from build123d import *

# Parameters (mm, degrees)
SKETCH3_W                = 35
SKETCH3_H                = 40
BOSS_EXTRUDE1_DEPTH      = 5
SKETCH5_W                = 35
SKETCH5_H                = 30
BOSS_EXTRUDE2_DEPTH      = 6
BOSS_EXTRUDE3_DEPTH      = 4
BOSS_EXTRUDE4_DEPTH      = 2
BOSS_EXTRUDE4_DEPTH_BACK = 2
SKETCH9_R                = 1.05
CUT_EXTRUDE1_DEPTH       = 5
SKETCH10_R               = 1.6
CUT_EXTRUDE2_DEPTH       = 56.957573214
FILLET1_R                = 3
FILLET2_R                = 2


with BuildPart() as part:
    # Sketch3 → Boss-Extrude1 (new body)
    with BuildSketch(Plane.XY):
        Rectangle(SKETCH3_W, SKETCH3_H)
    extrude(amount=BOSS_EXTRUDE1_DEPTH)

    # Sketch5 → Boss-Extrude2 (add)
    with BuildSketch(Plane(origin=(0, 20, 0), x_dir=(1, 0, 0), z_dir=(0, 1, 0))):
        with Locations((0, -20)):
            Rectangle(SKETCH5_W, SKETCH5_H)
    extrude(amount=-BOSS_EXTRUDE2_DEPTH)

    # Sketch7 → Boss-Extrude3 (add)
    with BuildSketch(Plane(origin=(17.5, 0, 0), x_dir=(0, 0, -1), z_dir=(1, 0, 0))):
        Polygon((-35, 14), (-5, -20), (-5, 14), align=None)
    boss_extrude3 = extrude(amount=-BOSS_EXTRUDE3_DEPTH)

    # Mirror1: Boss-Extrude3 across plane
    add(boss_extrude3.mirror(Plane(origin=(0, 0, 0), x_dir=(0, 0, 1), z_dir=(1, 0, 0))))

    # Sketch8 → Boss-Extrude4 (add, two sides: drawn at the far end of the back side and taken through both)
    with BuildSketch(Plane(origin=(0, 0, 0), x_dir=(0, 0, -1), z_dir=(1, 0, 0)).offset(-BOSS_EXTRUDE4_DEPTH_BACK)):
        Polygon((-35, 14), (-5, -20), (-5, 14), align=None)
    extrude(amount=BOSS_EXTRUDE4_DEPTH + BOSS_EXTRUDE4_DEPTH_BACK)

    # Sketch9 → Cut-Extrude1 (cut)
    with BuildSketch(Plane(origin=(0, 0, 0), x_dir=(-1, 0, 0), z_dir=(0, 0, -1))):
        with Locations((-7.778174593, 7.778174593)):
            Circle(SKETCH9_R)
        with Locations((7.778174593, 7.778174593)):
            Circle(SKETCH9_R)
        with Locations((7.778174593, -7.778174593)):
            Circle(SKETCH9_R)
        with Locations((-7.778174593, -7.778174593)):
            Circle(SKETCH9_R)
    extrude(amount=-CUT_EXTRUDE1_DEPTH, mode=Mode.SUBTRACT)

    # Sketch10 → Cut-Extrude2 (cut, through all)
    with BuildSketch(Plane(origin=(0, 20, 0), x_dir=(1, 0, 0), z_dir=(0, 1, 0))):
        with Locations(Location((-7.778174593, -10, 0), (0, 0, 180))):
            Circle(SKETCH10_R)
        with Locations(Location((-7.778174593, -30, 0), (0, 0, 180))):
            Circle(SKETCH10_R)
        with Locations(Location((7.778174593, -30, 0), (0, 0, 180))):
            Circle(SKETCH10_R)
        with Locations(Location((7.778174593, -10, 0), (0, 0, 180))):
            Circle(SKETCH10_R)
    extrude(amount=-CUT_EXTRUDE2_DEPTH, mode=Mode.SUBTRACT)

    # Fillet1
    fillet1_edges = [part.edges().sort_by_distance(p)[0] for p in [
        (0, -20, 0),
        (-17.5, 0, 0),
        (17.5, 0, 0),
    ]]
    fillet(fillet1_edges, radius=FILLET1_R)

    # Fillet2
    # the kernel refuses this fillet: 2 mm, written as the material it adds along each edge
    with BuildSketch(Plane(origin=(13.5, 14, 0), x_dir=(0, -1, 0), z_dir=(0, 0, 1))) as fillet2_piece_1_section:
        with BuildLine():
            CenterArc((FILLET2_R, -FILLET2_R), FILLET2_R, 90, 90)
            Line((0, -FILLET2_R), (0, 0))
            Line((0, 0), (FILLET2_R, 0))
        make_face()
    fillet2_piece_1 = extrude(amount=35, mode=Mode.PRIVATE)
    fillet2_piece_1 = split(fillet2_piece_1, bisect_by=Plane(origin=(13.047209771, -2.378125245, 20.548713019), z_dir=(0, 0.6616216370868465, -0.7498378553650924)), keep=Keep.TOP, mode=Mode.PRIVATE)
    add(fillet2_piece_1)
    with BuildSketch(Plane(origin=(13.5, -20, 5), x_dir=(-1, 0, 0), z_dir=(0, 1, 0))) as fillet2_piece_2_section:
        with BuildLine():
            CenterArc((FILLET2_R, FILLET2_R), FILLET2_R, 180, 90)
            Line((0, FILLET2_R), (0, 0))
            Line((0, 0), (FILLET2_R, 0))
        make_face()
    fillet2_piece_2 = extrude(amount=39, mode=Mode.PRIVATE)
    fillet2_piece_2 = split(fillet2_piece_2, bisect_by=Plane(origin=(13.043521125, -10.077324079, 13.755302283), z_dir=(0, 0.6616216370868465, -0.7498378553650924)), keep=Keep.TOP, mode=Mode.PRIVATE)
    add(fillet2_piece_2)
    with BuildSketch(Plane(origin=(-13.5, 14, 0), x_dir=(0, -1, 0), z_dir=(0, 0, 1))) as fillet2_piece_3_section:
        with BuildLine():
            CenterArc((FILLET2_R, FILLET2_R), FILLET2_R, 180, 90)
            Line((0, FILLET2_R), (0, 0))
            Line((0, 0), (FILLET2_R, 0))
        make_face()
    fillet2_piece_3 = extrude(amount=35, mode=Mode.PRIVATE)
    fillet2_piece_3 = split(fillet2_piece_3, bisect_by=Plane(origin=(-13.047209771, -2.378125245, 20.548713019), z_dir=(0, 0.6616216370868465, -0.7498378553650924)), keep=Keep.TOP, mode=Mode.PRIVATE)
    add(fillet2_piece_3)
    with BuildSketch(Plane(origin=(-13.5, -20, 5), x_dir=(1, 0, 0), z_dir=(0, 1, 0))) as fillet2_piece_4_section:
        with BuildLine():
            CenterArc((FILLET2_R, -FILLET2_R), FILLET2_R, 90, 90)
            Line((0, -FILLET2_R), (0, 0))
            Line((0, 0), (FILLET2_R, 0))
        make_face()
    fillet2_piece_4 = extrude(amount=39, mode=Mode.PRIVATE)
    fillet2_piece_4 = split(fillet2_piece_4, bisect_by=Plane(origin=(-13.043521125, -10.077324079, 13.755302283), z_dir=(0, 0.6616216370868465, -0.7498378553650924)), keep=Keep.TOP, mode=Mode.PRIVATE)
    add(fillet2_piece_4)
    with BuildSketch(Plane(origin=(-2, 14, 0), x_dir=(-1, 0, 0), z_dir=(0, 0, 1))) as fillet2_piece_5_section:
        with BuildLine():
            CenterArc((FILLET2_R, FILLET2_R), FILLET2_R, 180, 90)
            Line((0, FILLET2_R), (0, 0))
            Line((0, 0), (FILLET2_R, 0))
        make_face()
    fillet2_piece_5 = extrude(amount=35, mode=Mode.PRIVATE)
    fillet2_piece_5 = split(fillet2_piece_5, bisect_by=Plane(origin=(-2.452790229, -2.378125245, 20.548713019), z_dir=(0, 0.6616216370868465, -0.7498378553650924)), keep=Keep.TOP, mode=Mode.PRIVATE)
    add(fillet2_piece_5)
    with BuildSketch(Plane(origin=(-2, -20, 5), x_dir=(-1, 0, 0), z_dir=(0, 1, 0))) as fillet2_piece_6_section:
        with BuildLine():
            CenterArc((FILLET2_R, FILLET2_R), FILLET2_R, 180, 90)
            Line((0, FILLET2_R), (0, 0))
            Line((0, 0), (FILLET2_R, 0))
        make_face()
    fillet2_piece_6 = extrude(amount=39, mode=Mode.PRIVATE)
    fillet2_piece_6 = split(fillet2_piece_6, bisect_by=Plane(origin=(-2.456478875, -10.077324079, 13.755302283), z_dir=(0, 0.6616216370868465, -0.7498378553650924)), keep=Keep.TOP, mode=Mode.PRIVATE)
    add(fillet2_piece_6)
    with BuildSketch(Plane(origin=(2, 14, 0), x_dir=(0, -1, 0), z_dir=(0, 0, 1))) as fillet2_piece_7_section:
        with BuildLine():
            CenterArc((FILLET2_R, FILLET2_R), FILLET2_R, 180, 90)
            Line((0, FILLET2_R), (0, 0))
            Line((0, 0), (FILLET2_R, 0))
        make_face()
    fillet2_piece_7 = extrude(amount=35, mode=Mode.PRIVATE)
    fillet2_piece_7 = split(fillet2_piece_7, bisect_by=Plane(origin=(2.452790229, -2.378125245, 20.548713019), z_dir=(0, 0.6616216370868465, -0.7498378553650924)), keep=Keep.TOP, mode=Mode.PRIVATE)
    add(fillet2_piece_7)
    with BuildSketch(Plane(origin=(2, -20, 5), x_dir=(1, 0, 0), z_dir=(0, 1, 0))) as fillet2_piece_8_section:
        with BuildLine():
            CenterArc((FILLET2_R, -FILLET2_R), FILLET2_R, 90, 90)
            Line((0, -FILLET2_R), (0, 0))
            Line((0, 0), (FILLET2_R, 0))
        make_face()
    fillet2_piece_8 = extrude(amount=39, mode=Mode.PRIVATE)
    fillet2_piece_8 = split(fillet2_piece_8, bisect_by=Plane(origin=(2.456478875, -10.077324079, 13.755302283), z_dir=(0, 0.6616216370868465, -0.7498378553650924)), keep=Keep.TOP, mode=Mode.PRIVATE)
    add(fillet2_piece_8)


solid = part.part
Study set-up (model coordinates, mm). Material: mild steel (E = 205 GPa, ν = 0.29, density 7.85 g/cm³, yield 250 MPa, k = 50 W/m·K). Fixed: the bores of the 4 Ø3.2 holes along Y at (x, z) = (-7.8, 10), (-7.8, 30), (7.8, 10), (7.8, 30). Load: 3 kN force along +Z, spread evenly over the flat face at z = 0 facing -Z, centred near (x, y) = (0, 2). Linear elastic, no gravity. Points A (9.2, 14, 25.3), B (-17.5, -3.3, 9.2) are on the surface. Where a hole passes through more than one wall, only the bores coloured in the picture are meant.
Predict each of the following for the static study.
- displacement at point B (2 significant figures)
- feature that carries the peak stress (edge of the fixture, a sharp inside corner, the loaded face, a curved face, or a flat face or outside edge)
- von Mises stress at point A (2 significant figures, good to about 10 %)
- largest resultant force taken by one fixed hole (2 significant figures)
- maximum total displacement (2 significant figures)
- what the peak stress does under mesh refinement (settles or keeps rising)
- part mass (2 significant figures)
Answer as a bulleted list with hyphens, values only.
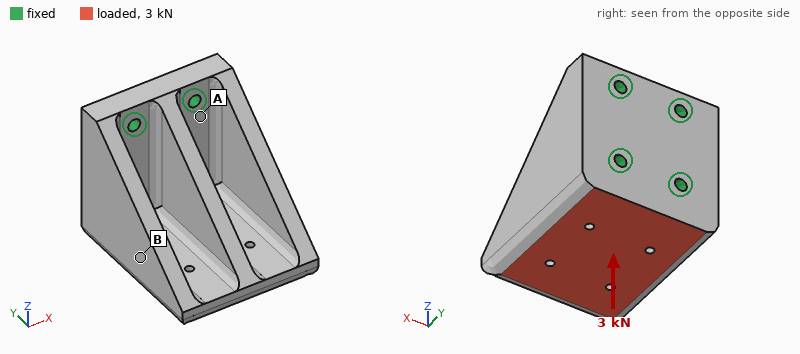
- 4.8 µm
- edge of the fixture
- 21 MPa
- 1.3 kN
- 12 µm
- keeps rising
- 150 g
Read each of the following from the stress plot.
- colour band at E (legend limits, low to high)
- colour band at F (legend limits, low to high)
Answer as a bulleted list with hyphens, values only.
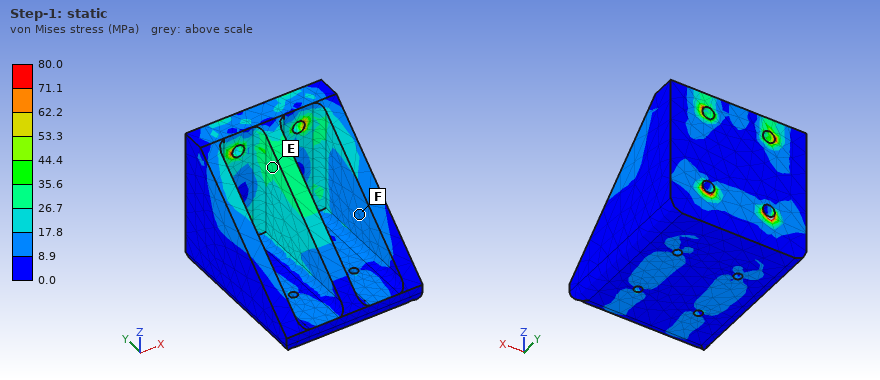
- 26.7 to 35.6 MPa
- 8.9 to 17.8 MPa
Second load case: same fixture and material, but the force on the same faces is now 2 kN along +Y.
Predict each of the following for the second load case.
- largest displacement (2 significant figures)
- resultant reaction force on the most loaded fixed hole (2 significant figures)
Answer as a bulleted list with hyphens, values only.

- 7.0 µm
- 1.3 kN
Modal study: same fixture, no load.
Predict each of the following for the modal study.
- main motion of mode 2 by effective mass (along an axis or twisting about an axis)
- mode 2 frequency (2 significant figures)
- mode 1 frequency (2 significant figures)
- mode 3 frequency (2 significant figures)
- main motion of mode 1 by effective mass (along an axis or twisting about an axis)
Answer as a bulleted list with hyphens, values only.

- along Z
- 10000 Hz
- 6900 Hz
- 15 kHz
- along X
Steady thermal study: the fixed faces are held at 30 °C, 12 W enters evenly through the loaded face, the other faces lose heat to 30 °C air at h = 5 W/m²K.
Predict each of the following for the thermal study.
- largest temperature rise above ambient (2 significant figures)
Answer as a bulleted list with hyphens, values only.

- 15 K
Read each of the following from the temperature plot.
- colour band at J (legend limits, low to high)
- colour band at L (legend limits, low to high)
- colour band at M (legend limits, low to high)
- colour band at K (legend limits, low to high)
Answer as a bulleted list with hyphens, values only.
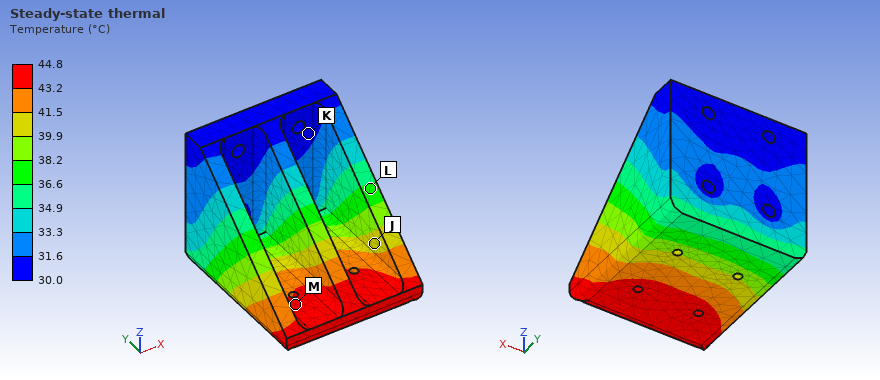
- 39.9 to 41.5 °C
- 36.6 to 38.2 °C
- 43.2 to 44.8 °C
- 30.0 to 31.6 °C
